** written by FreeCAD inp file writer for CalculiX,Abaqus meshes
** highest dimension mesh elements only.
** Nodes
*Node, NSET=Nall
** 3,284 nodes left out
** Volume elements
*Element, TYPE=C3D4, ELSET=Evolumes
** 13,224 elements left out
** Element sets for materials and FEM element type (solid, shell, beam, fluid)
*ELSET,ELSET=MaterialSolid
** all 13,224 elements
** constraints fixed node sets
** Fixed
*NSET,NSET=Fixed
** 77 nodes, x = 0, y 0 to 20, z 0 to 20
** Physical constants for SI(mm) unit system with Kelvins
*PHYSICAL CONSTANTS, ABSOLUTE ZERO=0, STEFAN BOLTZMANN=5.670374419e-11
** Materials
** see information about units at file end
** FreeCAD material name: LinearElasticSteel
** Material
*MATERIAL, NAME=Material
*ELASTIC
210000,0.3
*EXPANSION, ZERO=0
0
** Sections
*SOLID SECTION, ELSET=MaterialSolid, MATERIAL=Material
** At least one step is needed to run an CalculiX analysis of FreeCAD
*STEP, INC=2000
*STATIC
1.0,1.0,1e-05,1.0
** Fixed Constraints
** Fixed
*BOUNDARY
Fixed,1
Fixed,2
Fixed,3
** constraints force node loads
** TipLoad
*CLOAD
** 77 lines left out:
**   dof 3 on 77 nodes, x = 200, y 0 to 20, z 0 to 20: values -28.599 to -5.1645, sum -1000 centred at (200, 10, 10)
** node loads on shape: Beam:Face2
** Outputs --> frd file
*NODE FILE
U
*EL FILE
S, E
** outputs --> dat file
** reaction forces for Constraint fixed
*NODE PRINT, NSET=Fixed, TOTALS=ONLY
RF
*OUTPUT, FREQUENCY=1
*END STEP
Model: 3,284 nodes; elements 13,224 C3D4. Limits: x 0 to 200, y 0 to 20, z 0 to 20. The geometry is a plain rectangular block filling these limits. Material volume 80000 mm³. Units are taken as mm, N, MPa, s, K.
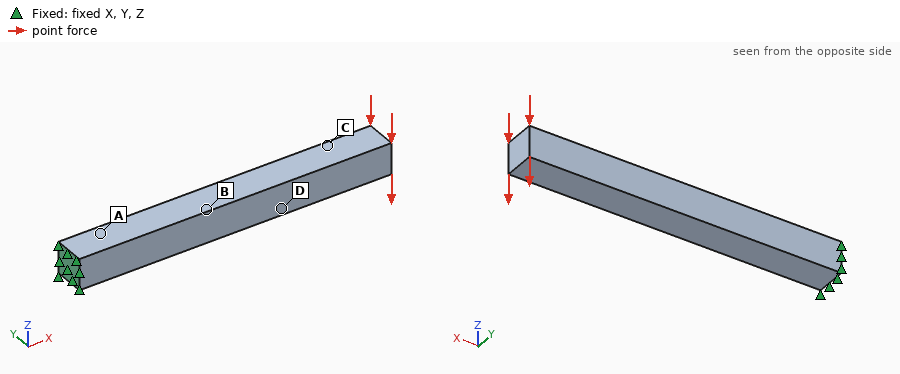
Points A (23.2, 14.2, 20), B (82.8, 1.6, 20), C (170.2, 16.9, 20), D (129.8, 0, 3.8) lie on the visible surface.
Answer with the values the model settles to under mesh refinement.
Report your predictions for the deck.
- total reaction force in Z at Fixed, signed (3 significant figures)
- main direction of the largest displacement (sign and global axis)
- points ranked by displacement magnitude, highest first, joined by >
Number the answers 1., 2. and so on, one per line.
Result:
1. 1000 N
2. -Z
3. C > D > B > A
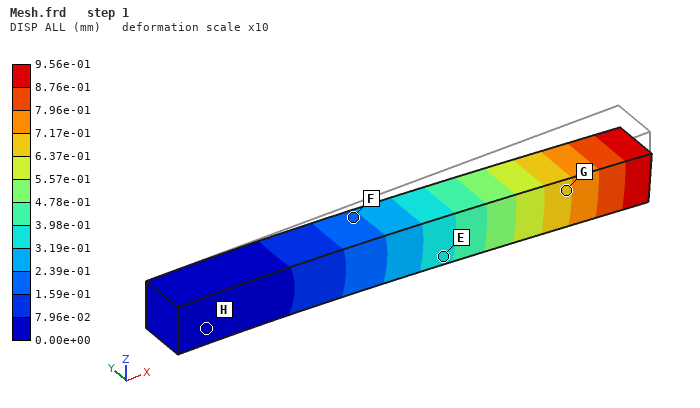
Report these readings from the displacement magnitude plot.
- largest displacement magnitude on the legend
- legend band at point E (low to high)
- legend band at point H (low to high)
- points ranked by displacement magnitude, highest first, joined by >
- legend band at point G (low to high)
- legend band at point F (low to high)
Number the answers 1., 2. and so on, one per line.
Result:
1. 9.56e-01 mm
2. 3.19e-01 to 3.98e-01 mm
3. 0.00e+00 to 7.96e-02 mm
4. G > E > F > H
5. 6.37e-01 to 7.17e-01 mm
6. 1.59e-01 to 2.39e-01 mm
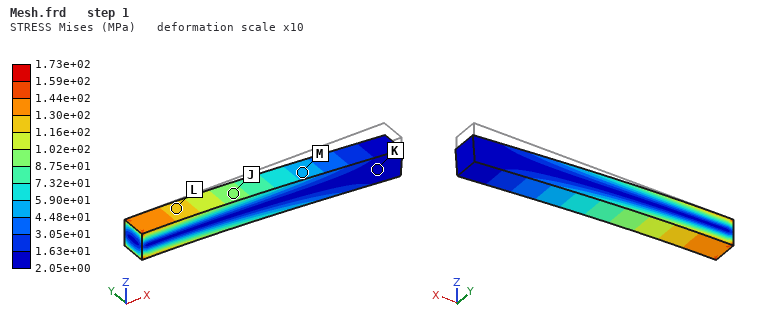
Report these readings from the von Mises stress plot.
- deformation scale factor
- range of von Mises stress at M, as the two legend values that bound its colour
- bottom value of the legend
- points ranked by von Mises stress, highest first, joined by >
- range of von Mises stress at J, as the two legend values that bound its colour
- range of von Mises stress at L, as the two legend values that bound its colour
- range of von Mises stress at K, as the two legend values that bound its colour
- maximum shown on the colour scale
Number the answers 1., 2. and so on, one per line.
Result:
1. 10
2. 4.48e+01 to 5.90e+01 MPa
3. 2.05e+00 MPa
4. L > J > M > K
5. 8.75e+01 to 1.02e+02 MPa
6. 1.16e+02 to 1.30e+02 MPa
7. 2.05e+00 to 1.63e+01 MPa
8. 1.73e+02 MPa
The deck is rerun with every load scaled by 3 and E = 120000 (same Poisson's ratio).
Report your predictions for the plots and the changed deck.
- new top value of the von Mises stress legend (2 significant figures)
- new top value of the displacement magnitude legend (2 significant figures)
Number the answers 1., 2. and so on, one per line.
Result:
1. 520 MPa
2. 5.0 mm
